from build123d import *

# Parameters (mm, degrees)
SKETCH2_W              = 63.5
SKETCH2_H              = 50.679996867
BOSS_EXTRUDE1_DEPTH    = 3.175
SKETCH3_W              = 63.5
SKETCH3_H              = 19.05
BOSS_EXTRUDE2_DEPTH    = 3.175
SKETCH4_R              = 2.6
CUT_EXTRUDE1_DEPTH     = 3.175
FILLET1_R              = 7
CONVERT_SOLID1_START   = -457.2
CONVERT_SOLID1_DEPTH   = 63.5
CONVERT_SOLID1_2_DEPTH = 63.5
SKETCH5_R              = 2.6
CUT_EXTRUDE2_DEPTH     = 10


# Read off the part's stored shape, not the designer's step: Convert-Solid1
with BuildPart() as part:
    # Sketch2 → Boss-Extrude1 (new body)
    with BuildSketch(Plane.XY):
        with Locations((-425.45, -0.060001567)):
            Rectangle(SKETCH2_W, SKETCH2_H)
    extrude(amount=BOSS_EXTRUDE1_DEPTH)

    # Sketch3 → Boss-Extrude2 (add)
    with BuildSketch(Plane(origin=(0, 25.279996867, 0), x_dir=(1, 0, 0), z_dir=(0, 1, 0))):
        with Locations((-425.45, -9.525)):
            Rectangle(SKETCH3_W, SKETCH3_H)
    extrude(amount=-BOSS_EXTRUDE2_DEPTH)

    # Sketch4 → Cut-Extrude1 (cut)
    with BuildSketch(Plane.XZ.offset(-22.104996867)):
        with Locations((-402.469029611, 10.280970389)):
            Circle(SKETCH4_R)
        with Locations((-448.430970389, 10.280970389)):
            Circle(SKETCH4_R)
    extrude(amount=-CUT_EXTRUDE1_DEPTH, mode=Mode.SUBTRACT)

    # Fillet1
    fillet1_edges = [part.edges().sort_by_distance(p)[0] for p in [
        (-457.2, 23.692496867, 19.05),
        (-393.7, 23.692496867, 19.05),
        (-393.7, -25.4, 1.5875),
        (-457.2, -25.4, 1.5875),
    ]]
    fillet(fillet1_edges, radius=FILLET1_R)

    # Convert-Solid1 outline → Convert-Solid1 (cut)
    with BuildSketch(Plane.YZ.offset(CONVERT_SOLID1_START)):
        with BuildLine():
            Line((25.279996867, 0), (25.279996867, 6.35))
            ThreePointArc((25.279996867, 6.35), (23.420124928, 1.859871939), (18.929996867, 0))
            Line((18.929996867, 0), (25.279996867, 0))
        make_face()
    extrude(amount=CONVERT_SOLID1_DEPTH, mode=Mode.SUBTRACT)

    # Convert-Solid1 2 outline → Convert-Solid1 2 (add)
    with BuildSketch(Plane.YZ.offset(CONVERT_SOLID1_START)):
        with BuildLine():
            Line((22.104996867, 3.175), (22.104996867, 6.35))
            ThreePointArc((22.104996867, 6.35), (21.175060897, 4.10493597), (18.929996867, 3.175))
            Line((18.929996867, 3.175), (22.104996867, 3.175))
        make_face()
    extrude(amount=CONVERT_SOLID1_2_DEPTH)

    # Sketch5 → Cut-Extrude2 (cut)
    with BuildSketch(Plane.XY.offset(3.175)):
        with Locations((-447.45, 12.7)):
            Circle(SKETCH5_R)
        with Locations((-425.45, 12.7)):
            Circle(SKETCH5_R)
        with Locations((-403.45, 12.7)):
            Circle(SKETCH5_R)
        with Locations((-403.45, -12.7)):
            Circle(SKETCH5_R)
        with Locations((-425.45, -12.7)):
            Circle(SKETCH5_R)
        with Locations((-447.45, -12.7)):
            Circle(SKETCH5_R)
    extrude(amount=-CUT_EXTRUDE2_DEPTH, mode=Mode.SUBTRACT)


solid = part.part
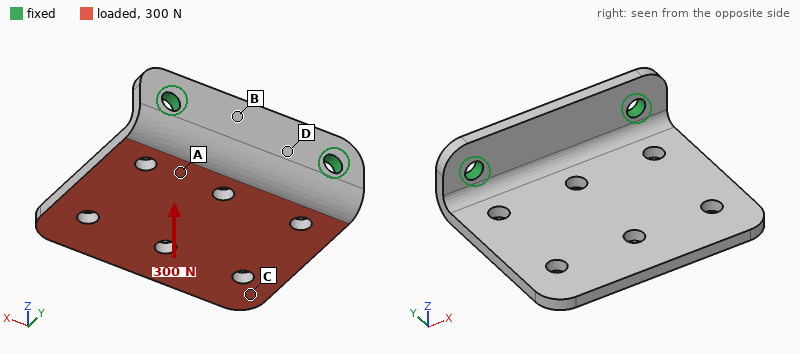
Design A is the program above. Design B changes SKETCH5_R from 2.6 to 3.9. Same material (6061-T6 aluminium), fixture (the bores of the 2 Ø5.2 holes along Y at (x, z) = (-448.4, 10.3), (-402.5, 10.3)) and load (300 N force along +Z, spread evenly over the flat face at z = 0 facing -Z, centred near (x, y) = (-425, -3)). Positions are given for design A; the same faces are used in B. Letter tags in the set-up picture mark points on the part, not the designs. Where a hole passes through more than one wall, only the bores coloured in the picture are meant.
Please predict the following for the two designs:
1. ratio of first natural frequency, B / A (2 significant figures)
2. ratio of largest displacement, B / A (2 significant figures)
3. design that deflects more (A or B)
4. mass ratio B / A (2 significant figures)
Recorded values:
0.99
1.1
B
0.96
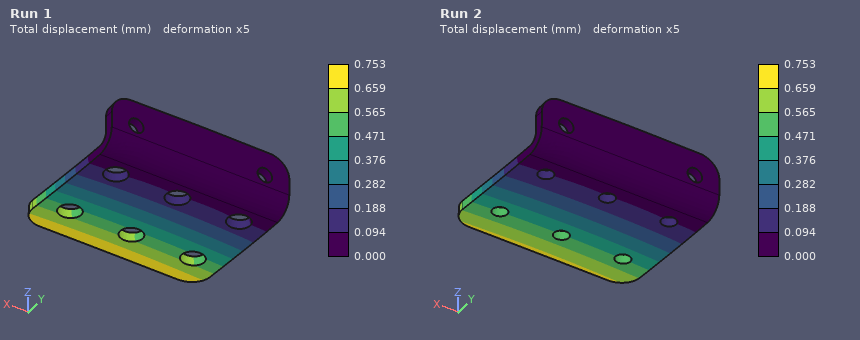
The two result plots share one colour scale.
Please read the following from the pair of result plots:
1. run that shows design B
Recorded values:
Run 1
